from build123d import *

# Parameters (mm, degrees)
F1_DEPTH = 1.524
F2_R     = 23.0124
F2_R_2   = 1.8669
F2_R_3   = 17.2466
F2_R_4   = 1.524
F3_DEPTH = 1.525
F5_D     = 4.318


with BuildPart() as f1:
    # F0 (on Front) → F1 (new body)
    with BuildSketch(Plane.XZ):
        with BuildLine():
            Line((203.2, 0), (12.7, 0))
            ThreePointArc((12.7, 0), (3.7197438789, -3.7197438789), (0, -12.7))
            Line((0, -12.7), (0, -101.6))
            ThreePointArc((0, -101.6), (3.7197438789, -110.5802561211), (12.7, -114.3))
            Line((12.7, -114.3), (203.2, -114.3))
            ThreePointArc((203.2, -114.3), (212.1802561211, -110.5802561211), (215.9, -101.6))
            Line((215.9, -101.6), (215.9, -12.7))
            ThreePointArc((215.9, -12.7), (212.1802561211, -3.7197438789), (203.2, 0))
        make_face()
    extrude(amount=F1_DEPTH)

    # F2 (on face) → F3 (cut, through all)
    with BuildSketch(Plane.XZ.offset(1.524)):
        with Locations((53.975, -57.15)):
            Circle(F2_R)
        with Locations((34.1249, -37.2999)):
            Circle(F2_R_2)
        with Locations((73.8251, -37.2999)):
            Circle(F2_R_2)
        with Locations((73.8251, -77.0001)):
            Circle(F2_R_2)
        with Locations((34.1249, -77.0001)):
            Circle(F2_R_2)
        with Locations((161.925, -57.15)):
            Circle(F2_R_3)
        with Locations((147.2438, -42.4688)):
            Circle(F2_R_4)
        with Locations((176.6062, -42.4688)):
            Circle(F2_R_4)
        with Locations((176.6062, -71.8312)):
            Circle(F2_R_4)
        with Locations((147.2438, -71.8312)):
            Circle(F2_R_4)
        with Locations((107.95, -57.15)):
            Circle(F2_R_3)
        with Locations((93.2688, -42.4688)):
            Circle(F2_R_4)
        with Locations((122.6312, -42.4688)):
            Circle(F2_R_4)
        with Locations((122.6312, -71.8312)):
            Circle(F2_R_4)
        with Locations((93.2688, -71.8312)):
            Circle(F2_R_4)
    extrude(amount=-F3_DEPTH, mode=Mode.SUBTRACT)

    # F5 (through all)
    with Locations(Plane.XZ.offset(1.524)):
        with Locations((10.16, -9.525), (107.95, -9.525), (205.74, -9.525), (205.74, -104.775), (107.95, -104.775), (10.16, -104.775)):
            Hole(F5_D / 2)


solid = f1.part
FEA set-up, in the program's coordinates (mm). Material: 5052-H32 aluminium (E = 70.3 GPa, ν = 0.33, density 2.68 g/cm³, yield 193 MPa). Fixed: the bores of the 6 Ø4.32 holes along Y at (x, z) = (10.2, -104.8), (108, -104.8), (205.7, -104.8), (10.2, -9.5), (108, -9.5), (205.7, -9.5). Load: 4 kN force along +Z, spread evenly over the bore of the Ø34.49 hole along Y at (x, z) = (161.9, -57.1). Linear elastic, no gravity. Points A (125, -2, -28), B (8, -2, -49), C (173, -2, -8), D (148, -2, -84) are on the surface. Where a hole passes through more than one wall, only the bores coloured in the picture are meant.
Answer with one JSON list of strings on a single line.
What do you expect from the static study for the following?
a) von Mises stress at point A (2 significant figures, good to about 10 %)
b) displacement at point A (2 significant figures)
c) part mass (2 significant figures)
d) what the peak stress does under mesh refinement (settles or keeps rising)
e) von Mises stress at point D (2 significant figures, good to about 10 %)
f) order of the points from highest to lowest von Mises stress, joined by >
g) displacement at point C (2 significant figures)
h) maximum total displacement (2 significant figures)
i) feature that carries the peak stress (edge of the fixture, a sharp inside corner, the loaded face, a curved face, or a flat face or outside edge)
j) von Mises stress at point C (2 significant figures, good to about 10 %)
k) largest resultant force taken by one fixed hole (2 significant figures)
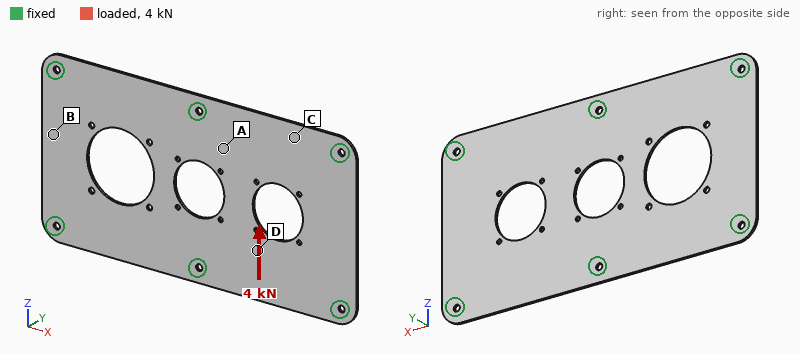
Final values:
["26 MPa", "17 µm", "85 g", "keeps rising", "18 MPa", "A > D > C > B", "25 µm", "34 µm", "edge of the fixture", "11 MPa", "1.2 kN"]
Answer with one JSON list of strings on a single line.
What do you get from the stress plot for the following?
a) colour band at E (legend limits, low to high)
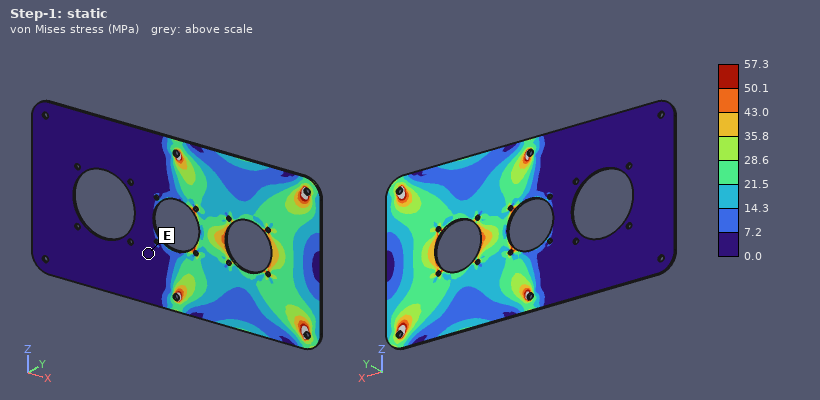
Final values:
["0.0 to 7.2 MPa"]
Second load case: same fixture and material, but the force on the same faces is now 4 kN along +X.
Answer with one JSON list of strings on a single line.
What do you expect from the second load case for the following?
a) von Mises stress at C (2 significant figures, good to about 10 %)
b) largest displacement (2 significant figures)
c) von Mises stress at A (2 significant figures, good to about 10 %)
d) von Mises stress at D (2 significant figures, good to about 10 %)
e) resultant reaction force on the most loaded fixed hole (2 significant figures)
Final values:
["9.4 MPa", "32 µm", "20 MPa", "25 MPa", "1.0 kN"]
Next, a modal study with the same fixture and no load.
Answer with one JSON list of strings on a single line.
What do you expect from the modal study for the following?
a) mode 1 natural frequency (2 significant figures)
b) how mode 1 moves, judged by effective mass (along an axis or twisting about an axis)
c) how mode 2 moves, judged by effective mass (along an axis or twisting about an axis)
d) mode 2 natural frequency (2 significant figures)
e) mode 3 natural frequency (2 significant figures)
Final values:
["600 Hz", "along Y", "along Y", "650 Hz", "900 Hz"]
